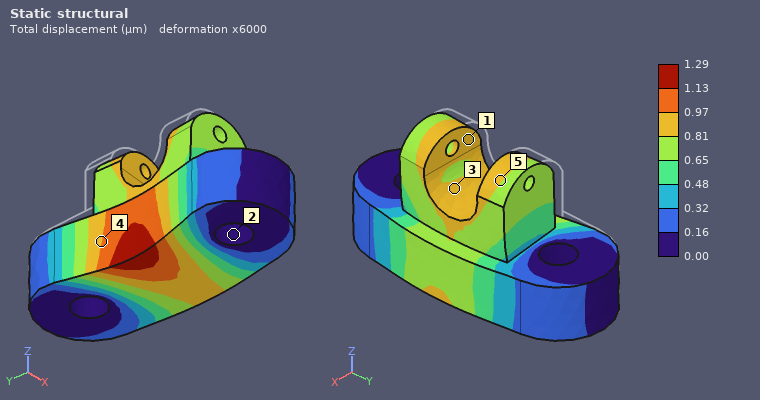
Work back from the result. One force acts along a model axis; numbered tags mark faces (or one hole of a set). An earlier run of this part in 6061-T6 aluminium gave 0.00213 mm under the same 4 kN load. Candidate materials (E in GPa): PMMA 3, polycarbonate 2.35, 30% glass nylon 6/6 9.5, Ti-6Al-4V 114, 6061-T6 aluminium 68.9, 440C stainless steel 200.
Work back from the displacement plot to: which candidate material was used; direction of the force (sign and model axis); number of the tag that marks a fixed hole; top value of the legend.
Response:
Ti-6Al-4V
+X
2
1.29 µm
